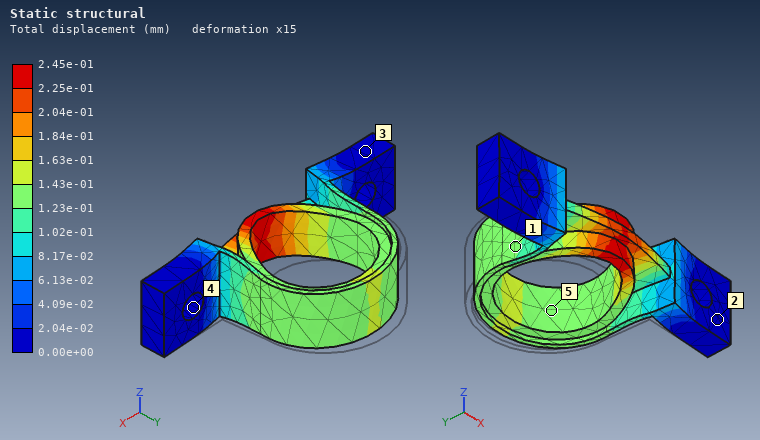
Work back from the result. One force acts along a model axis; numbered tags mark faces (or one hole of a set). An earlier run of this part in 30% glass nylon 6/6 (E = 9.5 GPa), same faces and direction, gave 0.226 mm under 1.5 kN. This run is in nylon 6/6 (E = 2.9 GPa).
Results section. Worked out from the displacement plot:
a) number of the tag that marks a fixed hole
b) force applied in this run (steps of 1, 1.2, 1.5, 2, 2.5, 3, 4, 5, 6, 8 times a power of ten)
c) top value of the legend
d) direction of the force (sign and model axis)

4
500 N
2.45e-01 mm
-Y
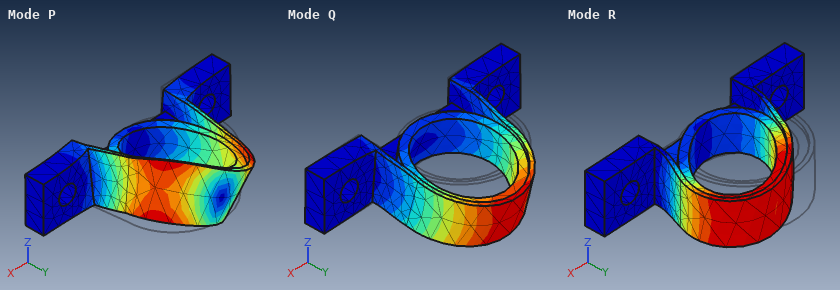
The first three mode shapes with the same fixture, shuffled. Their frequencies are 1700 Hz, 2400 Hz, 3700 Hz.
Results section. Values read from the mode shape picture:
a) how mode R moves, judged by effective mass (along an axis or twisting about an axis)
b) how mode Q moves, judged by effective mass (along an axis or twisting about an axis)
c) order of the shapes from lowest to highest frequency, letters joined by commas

along X
along Z
Q, R, P
